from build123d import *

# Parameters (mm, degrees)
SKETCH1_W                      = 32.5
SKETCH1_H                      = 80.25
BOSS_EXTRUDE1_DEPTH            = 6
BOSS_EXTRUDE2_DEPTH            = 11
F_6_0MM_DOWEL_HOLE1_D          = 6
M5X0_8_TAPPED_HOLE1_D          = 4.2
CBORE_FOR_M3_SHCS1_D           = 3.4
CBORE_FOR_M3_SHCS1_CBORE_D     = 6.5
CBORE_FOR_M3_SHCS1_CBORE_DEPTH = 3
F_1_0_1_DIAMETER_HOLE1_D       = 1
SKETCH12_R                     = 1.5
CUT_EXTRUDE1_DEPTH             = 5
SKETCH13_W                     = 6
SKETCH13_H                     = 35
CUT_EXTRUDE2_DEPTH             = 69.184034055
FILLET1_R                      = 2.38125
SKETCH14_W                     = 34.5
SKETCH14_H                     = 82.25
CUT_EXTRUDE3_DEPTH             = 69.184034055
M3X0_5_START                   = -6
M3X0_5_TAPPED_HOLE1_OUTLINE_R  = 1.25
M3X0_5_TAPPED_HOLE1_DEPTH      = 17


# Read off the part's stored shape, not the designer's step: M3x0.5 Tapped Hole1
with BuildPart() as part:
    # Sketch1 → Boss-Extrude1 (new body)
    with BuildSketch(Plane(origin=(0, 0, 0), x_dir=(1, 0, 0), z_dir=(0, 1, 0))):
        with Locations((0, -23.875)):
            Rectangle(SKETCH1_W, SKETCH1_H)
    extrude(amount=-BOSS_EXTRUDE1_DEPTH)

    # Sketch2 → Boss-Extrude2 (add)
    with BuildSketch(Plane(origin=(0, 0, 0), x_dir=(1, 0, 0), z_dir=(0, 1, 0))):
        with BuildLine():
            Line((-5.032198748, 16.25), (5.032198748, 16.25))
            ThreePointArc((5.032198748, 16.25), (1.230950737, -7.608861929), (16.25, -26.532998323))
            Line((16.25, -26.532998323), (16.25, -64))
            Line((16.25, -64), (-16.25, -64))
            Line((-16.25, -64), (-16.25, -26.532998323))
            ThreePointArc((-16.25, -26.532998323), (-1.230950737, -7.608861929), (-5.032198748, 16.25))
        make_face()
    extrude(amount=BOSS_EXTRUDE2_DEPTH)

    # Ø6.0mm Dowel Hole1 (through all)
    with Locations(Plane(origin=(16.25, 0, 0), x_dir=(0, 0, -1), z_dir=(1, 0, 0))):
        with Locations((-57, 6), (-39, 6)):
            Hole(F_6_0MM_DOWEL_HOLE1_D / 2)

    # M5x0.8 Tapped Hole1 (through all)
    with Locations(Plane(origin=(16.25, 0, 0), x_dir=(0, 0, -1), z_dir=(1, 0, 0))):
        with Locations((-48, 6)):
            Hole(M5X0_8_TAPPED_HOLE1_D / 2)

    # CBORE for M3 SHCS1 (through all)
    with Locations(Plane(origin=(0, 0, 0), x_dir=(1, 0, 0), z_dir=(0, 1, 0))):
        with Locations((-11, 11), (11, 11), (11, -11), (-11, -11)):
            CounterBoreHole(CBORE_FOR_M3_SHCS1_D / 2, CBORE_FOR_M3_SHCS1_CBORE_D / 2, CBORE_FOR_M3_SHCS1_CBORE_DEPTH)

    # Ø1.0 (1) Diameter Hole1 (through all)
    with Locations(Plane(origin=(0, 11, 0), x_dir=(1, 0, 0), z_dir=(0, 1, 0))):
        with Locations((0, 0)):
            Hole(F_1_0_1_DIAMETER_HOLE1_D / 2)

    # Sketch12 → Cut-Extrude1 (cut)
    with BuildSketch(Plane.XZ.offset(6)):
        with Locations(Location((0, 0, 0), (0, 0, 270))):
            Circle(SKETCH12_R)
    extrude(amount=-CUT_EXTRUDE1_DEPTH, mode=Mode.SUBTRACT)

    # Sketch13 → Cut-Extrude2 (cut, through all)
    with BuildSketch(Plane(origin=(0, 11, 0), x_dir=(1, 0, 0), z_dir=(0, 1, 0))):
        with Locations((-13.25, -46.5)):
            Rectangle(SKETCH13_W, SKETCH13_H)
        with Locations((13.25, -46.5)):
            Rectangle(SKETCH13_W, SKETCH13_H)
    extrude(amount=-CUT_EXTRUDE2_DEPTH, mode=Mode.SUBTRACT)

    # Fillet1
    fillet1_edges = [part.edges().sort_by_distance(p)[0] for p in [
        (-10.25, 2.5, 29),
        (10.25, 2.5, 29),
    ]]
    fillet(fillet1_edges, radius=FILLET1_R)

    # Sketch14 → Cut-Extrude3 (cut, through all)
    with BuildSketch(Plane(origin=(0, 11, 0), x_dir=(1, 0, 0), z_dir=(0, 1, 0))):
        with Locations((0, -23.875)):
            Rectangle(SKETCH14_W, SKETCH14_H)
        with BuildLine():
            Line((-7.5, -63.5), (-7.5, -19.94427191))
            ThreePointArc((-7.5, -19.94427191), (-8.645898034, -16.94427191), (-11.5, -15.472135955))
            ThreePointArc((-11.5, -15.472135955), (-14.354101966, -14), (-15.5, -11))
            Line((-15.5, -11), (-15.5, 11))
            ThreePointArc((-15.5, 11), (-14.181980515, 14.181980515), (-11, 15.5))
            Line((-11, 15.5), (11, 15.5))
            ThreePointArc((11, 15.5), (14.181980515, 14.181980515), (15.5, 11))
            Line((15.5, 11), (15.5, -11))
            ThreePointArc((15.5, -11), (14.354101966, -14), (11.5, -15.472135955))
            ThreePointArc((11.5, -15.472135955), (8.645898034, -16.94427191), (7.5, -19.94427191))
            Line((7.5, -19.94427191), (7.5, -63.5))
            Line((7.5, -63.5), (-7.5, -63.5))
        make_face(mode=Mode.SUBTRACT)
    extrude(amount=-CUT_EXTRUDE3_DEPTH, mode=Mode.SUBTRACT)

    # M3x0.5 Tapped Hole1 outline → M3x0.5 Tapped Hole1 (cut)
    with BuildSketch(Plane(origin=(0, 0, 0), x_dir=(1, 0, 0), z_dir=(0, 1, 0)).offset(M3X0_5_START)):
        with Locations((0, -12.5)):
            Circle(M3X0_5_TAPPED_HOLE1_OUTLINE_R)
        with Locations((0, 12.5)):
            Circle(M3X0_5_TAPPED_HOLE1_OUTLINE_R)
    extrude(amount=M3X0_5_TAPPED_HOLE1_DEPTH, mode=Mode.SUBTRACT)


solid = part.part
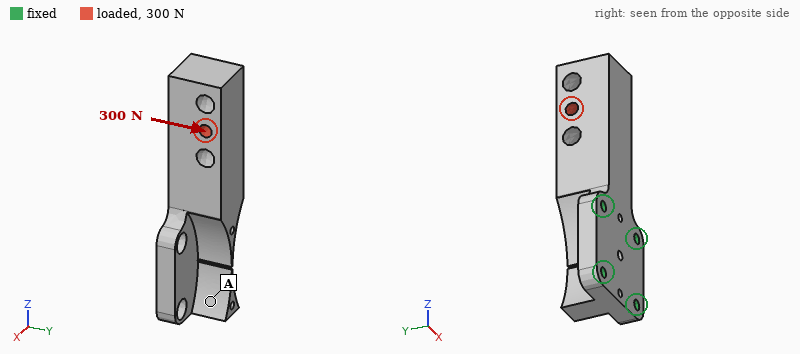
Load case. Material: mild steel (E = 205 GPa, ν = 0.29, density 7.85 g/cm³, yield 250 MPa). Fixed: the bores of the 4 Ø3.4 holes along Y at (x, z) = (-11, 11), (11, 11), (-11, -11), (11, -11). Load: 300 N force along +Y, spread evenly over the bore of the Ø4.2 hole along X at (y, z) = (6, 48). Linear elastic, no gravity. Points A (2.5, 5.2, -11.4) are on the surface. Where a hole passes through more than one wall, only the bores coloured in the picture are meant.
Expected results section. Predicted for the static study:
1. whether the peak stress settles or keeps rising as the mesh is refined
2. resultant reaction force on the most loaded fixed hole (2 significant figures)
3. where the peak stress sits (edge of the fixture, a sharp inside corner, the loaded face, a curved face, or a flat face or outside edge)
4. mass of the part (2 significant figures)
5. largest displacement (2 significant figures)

keeps rising
540 N
a sharp inside corner
130 g
46 µm
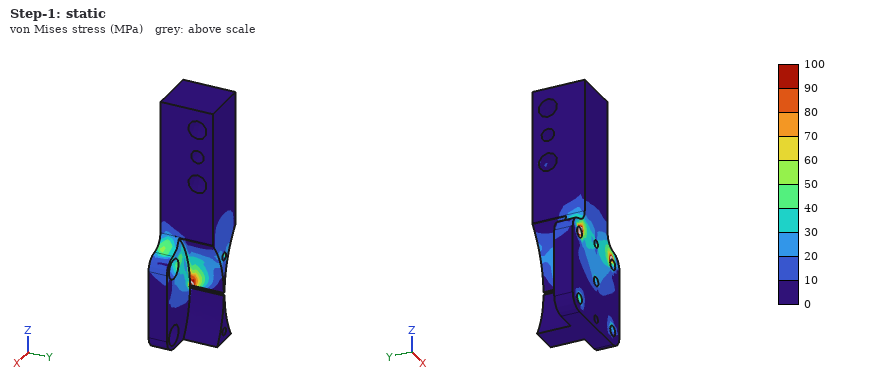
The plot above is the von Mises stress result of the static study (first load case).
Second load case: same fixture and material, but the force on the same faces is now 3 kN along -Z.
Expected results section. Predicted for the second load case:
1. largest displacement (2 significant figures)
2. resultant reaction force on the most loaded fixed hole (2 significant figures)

0.11 mm
1.3 kN
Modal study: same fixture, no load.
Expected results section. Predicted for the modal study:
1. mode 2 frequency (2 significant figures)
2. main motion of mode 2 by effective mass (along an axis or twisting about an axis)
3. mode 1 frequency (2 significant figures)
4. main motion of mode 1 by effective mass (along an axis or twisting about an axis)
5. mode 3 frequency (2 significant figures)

3500 Hz
along X
1900 Hz
along Y
9200 Hz
